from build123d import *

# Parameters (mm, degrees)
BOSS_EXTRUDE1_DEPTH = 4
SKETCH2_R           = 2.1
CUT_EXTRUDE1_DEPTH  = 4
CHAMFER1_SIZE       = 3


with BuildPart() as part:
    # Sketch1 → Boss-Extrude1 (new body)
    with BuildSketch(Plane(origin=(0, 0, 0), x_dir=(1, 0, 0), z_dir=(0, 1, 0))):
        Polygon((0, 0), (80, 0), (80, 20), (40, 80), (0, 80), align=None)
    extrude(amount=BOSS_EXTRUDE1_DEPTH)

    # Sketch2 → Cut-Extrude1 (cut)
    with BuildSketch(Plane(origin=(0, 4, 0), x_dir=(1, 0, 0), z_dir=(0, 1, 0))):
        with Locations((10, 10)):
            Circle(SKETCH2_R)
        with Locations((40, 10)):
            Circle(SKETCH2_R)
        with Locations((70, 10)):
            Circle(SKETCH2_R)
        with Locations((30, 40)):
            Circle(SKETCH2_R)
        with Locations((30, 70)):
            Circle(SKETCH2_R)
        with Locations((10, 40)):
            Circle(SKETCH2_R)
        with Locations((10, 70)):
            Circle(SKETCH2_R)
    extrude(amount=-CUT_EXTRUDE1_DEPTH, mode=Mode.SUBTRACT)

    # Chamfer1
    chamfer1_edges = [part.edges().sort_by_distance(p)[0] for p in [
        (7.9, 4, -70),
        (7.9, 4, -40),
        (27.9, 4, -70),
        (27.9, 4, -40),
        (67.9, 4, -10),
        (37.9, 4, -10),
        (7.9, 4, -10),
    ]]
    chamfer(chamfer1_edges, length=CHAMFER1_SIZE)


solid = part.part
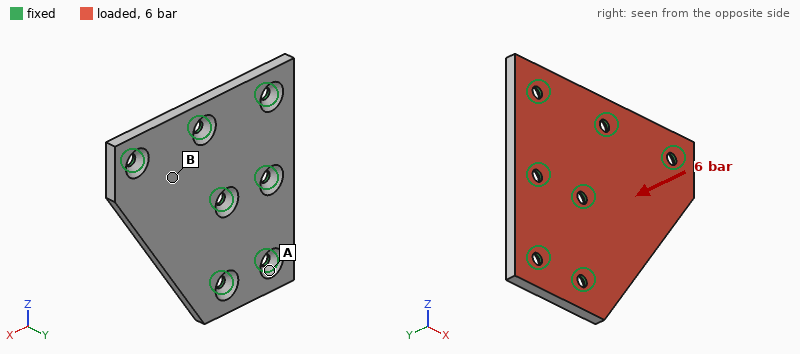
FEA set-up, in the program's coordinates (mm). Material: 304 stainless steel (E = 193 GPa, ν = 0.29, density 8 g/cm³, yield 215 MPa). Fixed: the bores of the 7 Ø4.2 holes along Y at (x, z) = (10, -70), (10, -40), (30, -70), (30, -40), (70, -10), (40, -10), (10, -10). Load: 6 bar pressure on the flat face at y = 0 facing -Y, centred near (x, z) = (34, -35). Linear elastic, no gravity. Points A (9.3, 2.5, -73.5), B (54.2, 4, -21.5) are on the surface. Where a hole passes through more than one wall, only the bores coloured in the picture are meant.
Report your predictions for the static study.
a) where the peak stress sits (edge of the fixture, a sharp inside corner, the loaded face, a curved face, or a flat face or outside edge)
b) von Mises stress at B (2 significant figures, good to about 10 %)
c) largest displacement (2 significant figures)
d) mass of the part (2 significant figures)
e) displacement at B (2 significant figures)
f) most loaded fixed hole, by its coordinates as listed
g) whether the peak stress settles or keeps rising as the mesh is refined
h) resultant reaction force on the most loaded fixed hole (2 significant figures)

edge of the fixture
31 MPa
50 µm
160 g
15 µm
(30, -40)
keeps rising
920 N
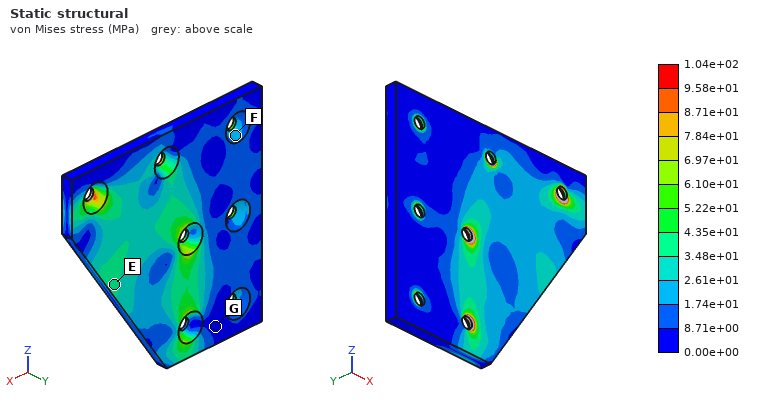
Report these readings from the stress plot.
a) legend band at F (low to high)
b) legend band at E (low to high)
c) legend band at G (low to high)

1.74e+01 to 2.61e+01 MPa
3.48e+01 to 4.35e+01 MPa
0.00e+00 to 8.71e+00 MPa
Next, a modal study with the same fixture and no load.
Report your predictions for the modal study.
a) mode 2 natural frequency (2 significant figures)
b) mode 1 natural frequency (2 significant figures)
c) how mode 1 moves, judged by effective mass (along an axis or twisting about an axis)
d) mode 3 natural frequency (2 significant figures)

8400 Hz
4100 Hz
along Y
12 kHz
